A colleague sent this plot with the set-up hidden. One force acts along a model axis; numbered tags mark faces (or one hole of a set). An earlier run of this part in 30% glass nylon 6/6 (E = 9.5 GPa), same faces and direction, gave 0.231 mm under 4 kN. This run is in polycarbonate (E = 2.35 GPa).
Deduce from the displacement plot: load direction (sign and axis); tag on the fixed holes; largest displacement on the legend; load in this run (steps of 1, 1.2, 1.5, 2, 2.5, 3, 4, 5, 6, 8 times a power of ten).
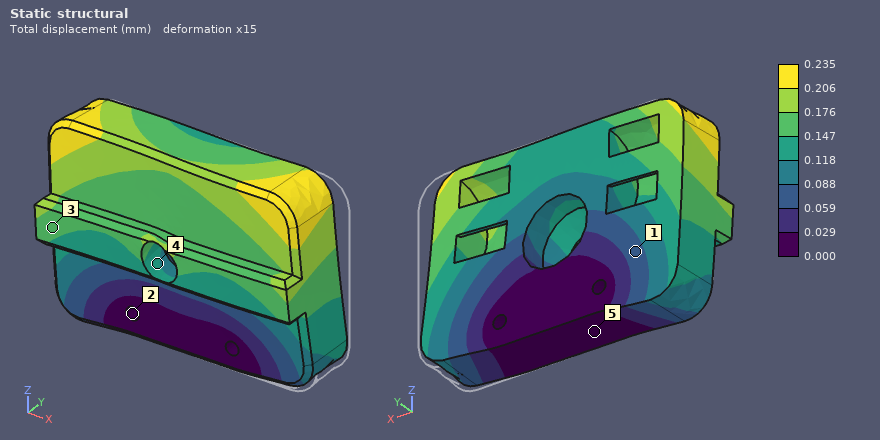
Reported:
-X
2
0.235 mm
1 kN
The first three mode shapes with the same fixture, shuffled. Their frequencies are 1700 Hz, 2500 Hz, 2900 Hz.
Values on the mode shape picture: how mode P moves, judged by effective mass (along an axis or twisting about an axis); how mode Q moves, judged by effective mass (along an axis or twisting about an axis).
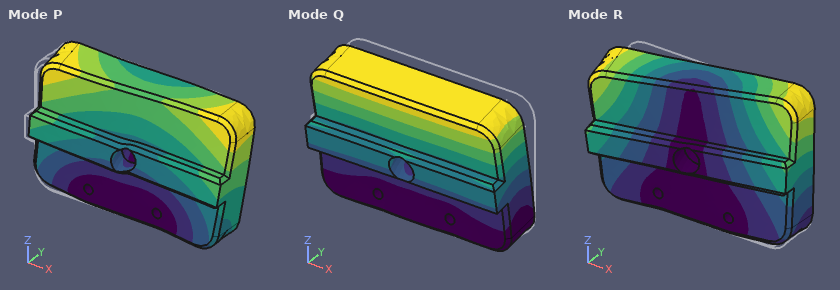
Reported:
along X
along Y
